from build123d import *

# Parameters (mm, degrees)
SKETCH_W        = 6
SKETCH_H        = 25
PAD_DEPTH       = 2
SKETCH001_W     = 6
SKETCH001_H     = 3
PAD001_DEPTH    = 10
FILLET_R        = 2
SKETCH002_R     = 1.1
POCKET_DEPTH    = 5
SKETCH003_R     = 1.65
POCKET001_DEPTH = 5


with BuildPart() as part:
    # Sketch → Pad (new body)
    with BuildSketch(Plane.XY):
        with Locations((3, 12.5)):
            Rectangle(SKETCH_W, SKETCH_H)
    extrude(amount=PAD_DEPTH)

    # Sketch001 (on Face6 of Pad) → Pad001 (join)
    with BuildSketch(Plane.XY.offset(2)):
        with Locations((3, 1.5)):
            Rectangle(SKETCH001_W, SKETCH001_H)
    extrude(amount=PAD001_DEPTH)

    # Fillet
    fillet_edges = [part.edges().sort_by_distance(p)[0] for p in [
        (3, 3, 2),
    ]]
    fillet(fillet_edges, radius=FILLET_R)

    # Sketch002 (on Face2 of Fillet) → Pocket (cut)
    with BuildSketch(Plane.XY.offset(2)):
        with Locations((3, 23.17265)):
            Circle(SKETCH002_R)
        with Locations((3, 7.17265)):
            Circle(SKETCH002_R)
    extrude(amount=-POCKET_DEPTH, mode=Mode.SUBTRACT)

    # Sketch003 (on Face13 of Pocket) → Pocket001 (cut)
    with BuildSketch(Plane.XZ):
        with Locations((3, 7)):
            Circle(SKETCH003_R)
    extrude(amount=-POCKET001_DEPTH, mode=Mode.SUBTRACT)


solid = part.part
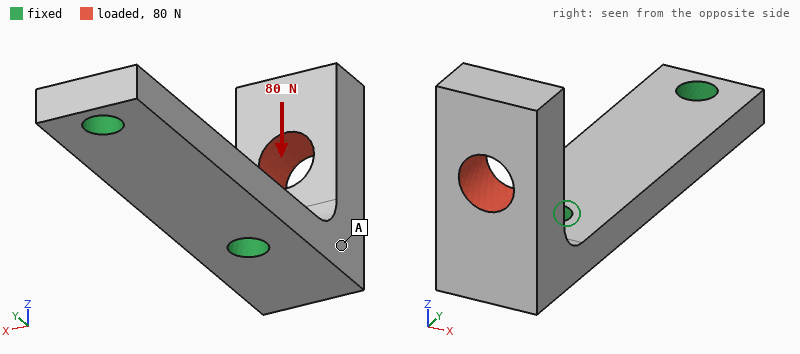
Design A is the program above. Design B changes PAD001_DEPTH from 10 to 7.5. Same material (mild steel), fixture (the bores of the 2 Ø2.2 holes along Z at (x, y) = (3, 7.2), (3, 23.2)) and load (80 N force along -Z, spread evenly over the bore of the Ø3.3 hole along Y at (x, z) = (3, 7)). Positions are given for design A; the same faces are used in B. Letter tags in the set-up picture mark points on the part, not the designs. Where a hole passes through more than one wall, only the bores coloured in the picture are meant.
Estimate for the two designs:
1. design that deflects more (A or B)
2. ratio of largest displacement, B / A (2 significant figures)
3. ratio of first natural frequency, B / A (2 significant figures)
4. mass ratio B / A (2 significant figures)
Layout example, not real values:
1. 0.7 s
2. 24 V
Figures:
1. A
2. 0.83
3. 1.5
4. 0.90
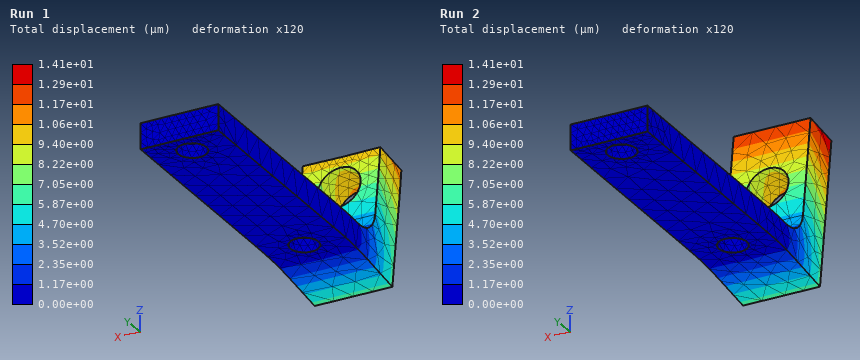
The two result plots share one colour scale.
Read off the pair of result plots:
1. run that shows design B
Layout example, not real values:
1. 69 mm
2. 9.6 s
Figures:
1. Run 1
